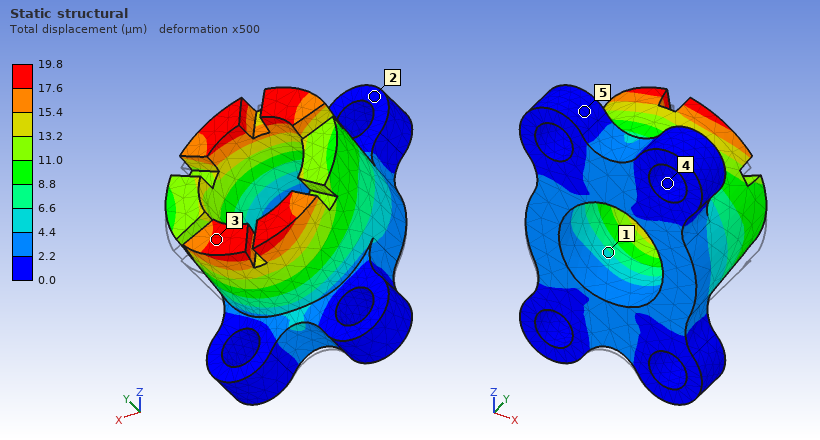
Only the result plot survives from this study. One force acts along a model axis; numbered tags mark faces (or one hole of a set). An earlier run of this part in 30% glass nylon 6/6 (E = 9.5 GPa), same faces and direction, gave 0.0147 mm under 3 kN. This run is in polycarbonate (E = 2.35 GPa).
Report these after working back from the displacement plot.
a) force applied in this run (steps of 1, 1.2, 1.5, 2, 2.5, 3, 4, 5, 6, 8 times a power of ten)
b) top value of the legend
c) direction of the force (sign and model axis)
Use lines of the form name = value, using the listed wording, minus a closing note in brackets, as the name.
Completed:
force applied in this run = 1 kN
top value of the legend = 19.8 µm
direction of the force = +Z
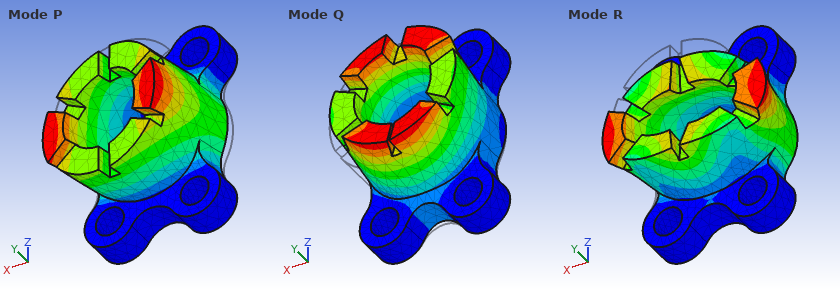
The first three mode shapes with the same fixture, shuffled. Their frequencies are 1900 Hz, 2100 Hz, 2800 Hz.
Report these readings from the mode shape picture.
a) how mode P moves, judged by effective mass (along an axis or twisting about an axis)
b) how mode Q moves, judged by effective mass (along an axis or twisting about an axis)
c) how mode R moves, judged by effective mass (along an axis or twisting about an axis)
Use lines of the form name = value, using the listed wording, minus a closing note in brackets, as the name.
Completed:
how mode P moves, judged by effective mass = along X
how mode Q moves, judged by effective mass = along Z
how mode R moves, judged by effective mass = along Y
